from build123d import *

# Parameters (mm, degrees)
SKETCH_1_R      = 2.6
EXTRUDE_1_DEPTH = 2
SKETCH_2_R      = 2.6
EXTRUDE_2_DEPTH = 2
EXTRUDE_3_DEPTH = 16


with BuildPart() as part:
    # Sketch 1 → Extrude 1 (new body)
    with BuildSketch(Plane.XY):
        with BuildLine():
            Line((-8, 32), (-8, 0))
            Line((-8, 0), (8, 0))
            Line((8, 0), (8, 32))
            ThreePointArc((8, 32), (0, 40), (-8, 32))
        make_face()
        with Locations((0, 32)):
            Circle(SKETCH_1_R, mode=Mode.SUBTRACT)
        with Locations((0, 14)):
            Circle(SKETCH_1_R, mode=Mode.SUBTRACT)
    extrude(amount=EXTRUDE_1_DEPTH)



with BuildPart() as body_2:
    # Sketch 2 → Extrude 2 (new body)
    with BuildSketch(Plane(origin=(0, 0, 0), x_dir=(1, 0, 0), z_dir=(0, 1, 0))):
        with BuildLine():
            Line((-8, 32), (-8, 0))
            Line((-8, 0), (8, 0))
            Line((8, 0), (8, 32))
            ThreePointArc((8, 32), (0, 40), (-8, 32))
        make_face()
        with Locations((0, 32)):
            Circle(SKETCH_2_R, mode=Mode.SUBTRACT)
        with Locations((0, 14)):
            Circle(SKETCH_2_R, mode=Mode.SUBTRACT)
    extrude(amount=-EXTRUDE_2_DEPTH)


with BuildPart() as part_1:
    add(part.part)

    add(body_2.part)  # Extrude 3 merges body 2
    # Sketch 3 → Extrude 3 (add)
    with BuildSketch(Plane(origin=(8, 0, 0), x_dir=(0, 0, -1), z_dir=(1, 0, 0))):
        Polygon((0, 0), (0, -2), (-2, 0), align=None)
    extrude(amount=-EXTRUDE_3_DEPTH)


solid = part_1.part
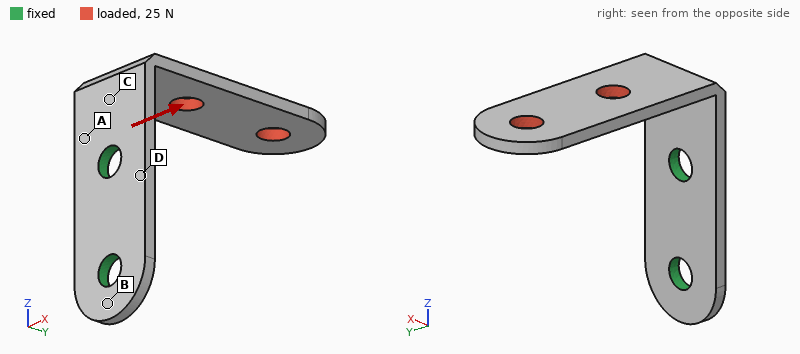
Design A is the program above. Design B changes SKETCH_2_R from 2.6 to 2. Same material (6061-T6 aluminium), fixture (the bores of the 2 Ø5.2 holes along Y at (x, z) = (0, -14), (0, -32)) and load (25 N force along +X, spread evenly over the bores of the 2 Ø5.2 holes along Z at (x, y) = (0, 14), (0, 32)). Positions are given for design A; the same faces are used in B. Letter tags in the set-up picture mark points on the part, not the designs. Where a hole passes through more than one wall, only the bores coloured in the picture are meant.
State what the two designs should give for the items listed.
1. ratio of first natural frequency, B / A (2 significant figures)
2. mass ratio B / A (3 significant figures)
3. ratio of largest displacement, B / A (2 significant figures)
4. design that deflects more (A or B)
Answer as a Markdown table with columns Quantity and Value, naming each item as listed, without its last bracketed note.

| Quantity | Value |
|---|---|
| ratio of first natural frequency, B / A | 0.98 |
| mass ratio B / A | 1.01 |
| ratio of largest displacement, B / A | 1.1 |
| design that deflects more | B |
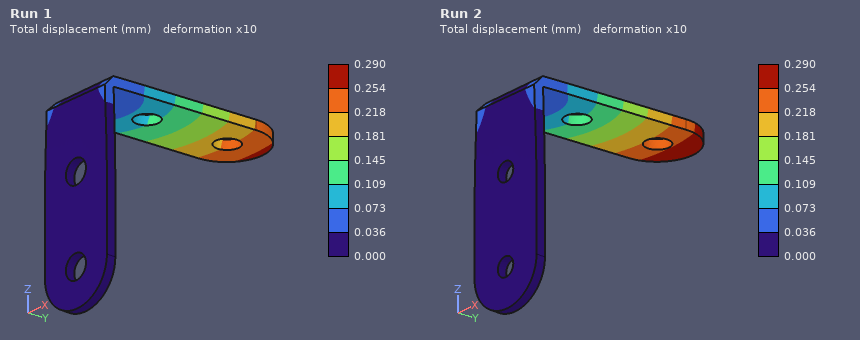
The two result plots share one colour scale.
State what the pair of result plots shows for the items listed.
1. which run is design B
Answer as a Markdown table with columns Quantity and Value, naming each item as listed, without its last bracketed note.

| Quantity | Value |
|---|---|
| which run is design B | Run 2 |
